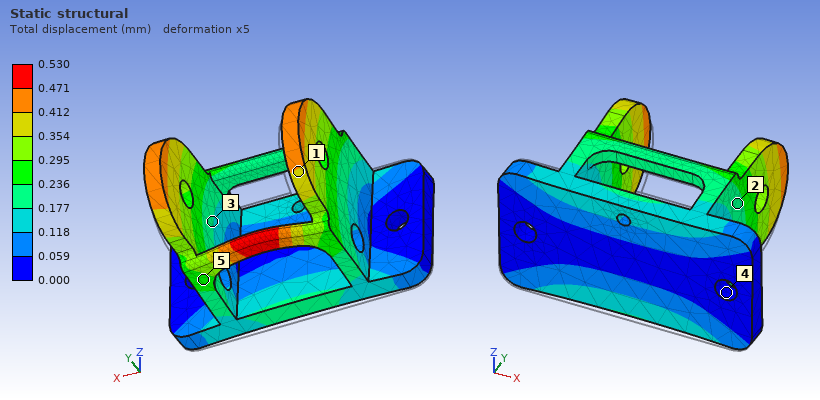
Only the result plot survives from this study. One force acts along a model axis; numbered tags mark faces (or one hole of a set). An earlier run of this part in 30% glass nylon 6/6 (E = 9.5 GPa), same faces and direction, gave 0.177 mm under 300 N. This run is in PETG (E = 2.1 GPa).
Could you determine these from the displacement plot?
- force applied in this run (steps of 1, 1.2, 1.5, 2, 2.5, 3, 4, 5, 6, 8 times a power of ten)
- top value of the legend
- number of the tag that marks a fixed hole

200 N
0.530 mm
4
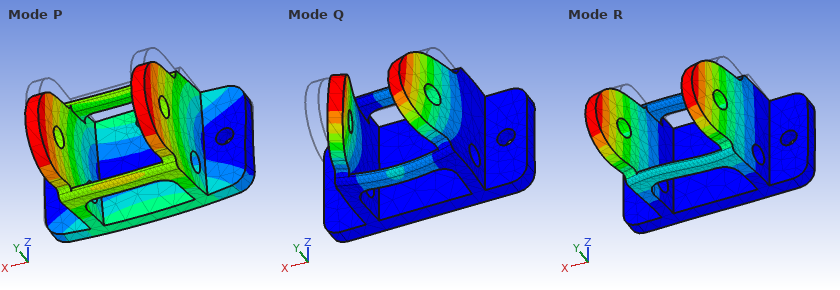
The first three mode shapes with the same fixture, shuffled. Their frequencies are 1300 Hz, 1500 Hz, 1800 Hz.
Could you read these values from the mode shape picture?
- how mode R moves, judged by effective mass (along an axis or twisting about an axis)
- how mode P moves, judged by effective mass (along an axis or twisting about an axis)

along X
along Z
